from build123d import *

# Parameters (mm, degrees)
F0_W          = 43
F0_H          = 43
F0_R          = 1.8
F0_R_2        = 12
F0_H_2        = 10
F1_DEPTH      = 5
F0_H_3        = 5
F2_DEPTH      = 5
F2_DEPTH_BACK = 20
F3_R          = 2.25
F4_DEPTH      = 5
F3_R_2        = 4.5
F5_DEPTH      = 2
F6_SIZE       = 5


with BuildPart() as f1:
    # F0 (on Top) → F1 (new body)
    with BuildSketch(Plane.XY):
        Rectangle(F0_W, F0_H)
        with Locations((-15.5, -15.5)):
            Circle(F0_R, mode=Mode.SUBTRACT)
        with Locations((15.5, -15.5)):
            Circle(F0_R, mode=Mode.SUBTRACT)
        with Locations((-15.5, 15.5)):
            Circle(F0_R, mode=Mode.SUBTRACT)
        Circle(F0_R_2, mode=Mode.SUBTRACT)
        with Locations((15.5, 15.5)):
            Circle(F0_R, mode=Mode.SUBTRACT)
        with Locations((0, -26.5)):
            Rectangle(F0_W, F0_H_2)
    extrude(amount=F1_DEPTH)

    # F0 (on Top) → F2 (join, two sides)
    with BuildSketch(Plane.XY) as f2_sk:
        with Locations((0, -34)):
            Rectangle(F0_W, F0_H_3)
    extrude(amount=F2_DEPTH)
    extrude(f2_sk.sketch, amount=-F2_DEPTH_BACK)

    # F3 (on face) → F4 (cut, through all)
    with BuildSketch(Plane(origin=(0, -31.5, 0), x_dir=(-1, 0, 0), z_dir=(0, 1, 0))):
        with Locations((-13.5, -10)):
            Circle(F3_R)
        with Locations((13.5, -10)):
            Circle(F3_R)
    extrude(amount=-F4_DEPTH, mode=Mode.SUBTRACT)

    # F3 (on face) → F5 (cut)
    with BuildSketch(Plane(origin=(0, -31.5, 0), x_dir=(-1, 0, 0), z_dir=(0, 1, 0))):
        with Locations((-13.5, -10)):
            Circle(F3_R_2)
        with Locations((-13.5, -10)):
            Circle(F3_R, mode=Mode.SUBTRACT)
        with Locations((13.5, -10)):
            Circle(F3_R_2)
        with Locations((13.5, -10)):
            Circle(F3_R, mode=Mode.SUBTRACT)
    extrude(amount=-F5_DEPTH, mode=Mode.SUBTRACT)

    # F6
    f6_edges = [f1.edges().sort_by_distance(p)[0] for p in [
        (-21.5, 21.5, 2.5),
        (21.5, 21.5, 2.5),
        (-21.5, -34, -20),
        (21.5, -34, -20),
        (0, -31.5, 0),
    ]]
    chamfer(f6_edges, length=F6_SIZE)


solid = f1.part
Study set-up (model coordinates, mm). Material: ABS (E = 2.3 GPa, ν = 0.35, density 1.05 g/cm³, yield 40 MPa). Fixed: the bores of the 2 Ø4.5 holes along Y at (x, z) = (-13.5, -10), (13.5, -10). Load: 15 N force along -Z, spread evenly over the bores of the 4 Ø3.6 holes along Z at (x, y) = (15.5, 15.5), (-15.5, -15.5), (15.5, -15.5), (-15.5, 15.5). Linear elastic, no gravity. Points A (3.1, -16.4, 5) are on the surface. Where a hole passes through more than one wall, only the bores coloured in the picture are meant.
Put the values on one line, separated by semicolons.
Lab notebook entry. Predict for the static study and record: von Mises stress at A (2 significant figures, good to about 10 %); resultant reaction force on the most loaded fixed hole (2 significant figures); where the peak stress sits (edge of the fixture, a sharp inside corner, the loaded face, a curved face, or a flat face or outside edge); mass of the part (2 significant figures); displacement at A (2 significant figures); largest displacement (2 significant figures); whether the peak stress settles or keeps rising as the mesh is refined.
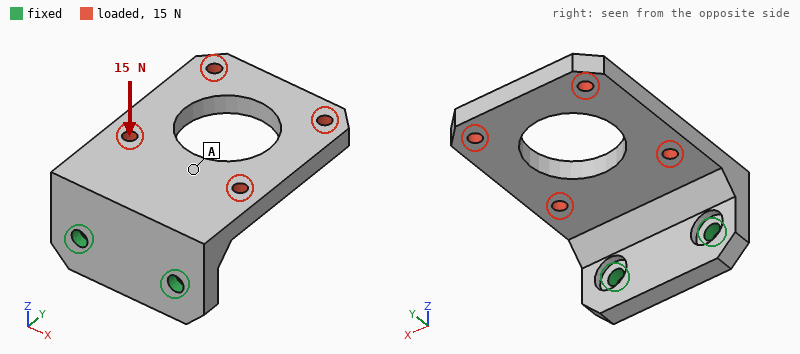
1.1 MPa; 7.9 N; edge of the fixture; 15 g; 0.18 mm; 0.77 mm; keeps rising
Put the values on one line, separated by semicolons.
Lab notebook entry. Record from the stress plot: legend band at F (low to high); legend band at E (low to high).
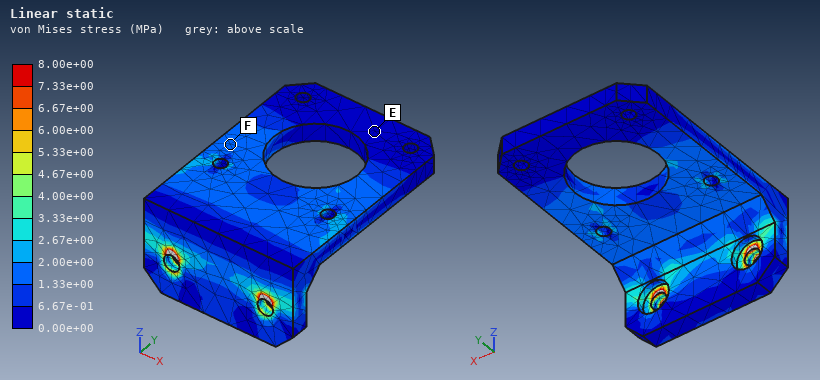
1.33e+00 to 2.00e+00 MPa; 0.00e+00 to 6.67e-01 MPa
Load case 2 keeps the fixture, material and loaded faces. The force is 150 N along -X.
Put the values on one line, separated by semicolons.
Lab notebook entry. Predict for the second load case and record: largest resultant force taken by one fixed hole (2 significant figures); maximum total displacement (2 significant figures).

210 N; 0.73 mm
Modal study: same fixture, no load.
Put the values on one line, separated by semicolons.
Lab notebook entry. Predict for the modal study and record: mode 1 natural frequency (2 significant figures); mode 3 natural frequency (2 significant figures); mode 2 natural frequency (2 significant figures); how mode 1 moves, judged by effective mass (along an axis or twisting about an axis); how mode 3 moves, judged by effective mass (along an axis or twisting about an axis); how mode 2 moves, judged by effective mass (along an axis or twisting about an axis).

320 Hz; 1200 Hz; 880 Hz; along Z; along X; along X
